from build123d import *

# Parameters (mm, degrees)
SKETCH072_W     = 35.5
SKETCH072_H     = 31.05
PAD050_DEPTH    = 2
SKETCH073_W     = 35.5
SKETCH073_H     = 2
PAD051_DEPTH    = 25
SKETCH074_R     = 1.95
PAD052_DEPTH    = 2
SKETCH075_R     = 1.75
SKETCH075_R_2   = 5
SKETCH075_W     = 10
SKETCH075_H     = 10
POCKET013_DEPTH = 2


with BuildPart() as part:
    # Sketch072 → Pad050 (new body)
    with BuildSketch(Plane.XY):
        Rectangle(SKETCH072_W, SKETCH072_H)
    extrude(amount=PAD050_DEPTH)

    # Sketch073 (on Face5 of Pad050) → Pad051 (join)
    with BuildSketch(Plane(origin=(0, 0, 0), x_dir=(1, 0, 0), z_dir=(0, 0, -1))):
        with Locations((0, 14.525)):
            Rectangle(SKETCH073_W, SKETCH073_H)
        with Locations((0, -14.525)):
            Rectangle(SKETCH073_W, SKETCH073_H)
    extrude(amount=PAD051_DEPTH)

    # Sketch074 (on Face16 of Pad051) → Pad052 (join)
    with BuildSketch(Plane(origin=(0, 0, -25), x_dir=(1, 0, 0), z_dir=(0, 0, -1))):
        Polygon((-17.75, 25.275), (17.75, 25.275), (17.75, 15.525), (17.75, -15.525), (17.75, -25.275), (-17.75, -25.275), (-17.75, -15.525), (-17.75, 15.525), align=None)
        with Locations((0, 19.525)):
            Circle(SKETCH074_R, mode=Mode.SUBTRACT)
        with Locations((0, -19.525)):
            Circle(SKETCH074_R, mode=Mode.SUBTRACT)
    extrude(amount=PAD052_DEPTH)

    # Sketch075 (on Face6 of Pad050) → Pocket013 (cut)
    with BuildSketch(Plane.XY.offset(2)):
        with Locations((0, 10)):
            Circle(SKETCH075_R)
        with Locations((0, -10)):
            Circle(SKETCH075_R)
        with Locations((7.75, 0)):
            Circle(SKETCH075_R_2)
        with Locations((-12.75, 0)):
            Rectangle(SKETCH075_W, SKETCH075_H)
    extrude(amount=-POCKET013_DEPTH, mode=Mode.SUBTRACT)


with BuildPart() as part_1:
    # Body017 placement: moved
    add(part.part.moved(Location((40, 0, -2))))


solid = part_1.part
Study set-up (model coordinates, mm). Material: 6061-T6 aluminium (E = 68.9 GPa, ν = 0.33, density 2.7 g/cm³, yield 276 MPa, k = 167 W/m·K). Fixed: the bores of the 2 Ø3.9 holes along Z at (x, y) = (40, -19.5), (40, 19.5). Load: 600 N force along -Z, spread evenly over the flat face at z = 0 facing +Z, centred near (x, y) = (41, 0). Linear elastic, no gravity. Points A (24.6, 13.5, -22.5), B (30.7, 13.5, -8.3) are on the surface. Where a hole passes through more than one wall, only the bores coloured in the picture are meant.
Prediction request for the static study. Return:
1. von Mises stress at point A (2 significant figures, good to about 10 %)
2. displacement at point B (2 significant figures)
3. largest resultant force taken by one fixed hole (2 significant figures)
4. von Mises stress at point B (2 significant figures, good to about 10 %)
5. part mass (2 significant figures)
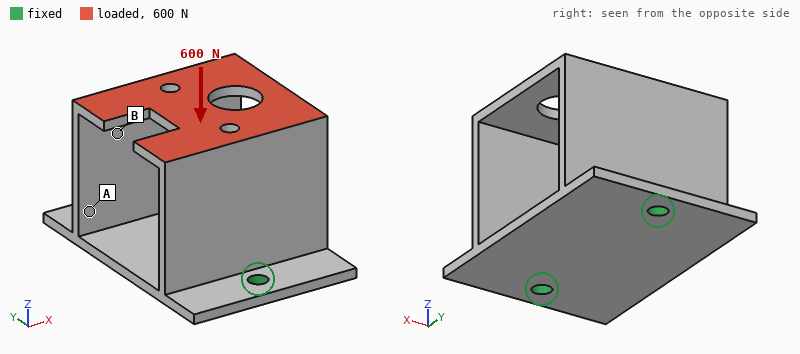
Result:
7.1 MPa
17 µm
310 N
28 MPa
24 g
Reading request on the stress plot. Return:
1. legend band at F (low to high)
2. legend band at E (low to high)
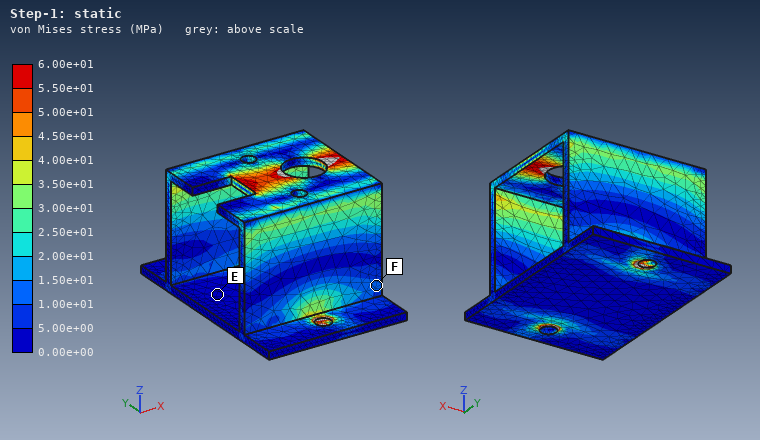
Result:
1.00e+01 to 1.50e+01 MPa
0.00e+00 to 5.00e+00 MPa
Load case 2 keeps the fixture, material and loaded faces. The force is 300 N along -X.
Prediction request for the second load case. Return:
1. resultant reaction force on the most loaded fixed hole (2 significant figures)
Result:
150 N
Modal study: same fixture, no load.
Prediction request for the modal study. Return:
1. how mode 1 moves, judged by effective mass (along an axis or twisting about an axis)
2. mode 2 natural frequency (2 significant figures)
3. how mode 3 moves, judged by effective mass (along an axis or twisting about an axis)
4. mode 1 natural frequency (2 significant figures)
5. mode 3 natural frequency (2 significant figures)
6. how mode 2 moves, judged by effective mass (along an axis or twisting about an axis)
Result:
along X
2000 Hz
twisting about Z
1700 Hz
3200 Hz
along Y
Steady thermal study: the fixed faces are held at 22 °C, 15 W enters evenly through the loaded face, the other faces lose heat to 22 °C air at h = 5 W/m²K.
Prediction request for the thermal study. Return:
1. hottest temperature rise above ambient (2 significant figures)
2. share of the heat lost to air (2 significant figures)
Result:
27 K
3.5 %
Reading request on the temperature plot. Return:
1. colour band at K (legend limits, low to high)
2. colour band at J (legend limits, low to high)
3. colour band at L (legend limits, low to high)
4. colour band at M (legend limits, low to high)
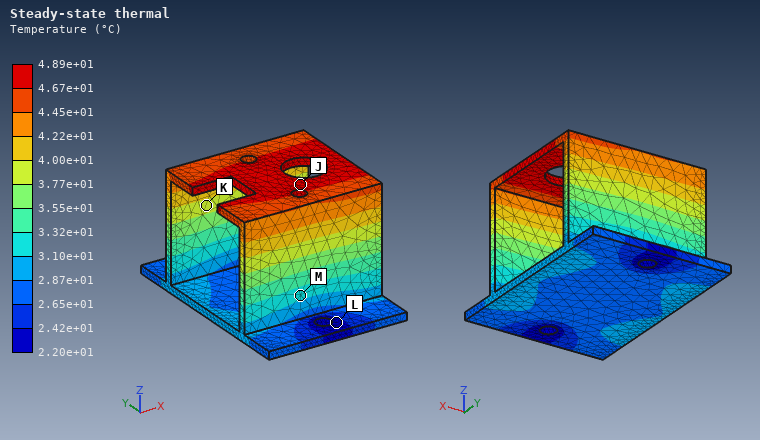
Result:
3.77e+01 to 4.00e+01 °C
4.67e+01 to 4.89e+01 °C
2.20e+01 to 2.42e+01 °C
3.10e+01 to 3.32e+01 °C
